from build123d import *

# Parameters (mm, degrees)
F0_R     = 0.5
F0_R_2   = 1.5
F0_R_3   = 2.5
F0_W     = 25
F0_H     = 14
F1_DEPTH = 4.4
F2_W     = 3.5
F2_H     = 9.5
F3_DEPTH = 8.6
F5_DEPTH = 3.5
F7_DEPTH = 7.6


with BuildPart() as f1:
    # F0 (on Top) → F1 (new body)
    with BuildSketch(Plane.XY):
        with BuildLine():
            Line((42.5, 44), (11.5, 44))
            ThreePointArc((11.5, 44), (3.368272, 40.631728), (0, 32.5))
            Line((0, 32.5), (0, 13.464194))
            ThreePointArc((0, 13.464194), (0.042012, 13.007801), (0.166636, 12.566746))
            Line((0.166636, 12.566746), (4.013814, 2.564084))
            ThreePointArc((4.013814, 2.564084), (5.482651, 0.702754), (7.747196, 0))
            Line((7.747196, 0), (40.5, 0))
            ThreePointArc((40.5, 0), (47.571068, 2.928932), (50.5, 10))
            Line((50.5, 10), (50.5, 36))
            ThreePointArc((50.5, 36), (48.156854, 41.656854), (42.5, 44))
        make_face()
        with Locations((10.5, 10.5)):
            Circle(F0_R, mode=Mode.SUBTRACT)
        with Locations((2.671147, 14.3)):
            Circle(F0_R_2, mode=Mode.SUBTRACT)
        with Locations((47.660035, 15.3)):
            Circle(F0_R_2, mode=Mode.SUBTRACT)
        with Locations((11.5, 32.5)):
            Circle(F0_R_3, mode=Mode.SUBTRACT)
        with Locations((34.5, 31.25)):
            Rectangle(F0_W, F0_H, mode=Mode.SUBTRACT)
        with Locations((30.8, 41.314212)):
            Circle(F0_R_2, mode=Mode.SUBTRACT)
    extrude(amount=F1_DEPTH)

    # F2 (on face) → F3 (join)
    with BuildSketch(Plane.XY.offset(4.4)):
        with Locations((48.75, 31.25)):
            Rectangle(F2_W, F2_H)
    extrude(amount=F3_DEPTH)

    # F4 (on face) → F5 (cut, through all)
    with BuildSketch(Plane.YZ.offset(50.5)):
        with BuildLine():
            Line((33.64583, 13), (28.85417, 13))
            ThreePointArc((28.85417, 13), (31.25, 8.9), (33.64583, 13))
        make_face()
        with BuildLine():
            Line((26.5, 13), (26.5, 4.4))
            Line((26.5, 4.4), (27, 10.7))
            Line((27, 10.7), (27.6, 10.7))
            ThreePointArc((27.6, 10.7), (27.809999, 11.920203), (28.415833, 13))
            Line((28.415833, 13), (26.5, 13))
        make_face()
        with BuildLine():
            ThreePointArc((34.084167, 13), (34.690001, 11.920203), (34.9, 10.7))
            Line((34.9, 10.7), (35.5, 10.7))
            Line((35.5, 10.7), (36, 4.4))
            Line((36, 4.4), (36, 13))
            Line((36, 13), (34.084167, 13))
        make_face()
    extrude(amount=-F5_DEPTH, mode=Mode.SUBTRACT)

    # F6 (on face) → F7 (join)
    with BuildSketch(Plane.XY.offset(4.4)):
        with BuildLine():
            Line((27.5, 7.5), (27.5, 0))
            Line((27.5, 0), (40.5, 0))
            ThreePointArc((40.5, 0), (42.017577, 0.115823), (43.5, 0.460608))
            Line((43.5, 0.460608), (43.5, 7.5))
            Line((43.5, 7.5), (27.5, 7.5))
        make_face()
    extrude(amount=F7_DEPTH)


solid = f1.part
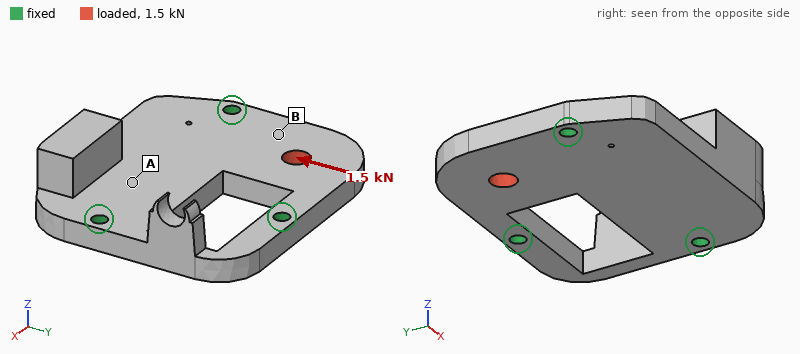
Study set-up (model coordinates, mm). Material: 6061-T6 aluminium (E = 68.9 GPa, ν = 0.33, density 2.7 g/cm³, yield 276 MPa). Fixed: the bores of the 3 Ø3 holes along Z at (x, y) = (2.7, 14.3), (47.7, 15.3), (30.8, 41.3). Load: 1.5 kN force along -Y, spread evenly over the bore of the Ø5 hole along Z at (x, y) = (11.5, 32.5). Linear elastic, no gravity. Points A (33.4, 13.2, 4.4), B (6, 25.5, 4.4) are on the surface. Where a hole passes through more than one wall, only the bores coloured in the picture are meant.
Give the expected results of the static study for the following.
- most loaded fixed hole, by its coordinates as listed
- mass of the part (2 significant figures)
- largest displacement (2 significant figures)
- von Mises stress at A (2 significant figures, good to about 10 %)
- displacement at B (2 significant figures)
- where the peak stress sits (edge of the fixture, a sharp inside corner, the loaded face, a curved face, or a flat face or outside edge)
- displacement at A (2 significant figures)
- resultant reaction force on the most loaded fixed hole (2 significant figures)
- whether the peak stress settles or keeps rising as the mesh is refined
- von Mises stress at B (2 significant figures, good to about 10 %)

(2.7, 14.3)
24 g
8.7 µm
4.9 MPa
4.3 µm
edge of the fixture
3.1 µm
1.2 kN
keeps rising
20 MPa
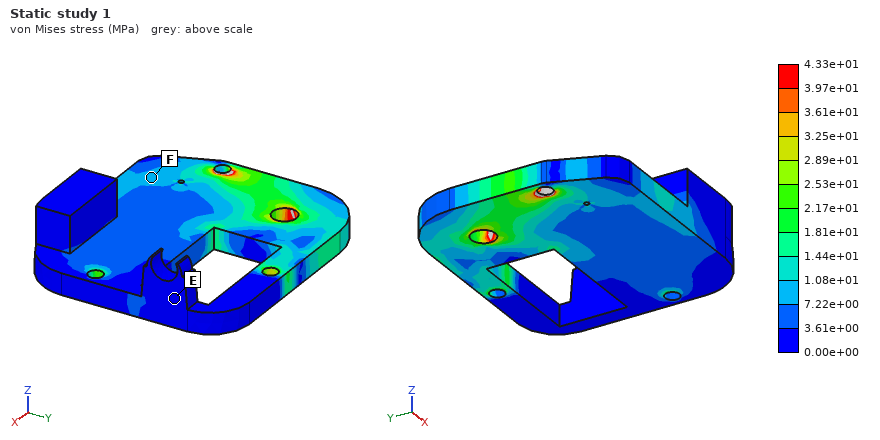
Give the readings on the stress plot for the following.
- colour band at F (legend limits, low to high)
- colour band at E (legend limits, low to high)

7.22e+00 to 1.08e+01 MPa
0.00e+00 to 3.61e+00 MPa
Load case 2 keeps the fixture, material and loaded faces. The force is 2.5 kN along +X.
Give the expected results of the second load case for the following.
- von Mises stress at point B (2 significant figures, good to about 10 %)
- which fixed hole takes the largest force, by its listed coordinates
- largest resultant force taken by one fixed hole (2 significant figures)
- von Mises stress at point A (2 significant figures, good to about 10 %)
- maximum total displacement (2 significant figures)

21 MPa
(30.8, 41.3)
1.2 kN
8.5 MPa
15 µm
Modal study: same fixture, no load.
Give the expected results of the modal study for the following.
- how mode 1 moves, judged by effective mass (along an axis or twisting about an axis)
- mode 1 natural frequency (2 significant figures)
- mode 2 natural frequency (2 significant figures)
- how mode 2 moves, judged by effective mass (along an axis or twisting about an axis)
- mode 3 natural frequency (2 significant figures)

along Z
6300 Hz
7900 Hz
along Z
10 kHz
